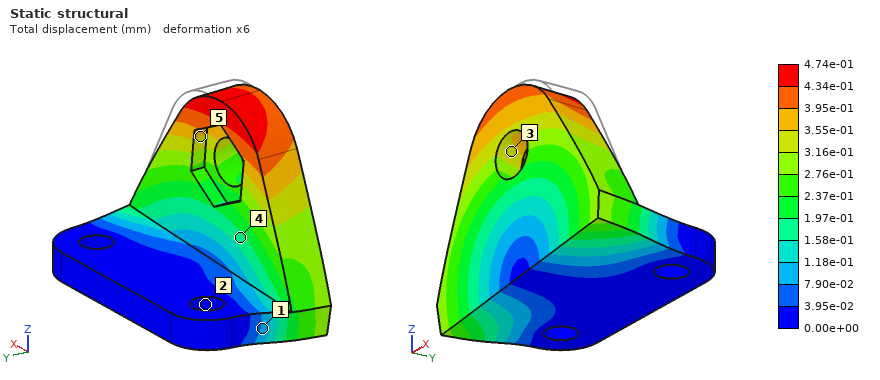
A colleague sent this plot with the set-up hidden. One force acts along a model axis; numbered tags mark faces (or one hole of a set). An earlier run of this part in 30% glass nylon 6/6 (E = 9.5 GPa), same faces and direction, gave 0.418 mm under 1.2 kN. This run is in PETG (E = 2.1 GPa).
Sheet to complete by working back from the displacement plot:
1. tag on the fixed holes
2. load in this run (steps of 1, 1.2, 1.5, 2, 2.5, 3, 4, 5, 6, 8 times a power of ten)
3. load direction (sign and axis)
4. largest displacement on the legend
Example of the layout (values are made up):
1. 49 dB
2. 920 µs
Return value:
1. 2
2. 300 N
3. -X
4. 4.74e-01 mm
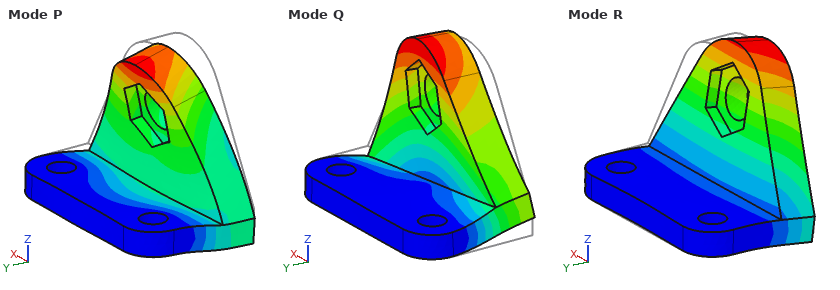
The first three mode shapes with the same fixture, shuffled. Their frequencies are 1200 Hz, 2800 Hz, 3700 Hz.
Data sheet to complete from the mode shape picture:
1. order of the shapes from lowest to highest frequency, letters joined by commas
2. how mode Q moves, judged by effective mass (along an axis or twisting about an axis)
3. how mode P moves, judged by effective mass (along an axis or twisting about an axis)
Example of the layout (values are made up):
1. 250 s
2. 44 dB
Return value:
1. R, Q, P
2. along X
3. along Z
